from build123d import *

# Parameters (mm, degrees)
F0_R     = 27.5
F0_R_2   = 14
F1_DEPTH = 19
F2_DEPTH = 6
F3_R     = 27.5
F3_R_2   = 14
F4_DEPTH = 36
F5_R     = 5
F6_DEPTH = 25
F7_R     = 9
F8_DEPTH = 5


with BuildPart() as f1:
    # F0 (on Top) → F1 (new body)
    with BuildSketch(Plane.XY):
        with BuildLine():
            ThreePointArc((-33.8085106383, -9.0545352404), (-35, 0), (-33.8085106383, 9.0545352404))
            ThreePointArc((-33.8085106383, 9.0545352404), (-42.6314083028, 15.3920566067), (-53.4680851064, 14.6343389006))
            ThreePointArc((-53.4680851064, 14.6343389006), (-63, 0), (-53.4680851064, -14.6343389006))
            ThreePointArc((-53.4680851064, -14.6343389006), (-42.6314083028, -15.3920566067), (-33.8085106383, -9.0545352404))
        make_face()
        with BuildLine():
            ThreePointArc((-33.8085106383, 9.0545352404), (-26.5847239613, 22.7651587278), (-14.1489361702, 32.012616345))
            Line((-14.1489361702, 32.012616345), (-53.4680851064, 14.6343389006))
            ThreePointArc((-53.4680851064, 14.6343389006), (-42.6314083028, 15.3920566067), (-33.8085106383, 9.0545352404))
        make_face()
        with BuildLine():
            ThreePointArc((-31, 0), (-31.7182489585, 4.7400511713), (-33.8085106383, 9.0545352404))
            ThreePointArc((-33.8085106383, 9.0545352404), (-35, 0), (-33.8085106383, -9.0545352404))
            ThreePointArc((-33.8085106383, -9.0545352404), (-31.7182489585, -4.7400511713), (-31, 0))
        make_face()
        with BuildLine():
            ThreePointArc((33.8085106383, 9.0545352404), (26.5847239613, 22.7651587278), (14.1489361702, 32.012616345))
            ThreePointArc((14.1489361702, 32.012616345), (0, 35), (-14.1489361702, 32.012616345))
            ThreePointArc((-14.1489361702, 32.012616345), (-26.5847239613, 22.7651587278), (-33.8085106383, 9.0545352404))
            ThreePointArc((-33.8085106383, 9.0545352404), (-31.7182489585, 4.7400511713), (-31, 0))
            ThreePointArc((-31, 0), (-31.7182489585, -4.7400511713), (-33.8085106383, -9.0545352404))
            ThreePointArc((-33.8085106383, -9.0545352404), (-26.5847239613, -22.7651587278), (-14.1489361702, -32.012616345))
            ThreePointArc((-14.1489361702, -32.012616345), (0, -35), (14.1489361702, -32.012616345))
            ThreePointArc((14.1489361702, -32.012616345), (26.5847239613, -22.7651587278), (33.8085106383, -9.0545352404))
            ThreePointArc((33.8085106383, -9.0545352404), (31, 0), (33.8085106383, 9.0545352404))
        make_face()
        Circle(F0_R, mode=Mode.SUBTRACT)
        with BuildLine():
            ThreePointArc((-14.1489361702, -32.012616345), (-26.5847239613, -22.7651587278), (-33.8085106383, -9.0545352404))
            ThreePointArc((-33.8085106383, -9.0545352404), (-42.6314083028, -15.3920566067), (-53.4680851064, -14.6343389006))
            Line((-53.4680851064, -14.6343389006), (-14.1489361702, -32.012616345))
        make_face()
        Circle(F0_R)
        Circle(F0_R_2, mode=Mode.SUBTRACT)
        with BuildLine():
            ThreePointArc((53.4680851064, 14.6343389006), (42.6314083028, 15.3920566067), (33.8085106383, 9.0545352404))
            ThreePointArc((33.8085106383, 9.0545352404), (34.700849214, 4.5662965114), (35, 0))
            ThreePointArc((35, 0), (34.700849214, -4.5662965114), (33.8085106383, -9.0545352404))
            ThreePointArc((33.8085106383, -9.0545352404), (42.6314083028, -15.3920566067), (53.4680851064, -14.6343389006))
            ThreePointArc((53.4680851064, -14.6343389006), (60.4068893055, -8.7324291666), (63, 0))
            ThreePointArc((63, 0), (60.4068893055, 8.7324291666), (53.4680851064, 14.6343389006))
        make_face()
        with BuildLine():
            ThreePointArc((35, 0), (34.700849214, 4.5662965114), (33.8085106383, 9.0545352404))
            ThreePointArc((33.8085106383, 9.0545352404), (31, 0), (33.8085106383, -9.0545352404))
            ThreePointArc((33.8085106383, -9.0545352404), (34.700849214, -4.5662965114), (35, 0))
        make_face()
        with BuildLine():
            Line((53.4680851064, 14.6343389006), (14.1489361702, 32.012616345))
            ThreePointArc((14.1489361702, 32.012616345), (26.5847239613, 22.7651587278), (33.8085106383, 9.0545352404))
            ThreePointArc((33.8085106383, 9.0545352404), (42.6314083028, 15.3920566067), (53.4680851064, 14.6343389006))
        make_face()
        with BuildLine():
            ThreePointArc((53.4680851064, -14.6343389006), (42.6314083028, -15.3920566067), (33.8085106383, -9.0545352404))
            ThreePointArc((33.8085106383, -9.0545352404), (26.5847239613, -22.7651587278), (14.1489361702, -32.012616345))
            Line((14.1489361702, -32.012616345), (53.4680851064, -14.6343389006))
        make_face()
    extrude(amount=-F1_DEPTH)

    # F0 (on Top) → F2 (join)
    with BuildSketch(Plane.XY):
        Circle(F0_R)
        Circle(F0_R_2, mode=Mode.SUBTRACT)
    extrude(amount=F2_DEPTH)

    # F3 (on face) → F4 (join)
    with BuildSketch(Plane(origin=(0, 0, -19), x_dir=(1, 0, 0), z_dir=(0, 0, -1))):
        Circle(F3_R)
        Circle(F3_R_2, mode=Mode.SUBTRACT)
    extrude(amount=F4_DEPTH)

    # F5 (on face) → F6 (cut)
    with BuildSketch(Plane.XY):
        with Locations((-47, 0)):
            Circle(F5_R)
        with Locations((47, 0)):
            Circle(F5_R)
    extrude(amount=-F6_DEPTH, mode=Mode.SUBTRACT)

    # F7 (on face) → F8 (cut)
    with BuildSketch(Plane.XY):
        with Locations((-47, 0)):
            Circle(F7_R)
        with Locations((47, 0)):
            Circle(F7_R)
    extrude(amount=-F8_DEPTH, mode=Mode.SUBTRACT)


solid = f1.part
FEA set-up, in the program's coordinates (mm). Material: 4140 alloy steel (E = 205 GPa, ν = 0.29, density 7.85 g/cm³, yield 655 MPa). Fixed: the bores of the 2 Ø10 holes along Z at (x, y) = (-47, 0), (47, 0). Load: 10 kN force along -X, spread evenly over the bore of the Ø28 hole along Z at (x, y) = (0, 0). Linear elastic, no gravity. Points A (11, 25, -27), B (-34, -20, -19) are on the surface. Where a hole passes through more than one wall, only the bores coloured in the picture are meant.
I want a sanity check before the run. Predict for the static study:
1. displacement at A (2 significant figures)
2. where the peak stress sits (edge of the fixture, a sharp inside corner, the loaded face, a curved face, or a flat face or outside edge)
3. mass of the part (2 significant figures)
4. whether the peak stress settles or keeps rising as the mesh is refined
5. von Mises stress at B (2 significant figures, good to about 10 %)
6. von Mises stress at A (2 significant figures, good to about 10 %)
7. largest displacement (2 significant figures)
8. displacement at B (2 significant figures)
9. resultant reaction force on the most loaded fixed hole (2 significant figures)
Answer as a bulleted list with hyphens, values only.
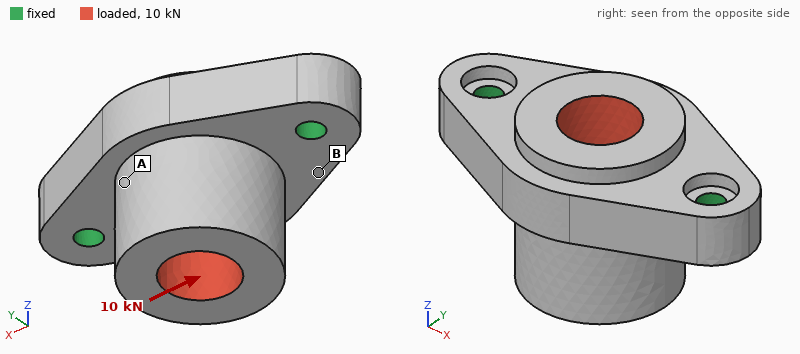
- 2.7 µm
- edge of the fixture
- 1.3 kg
- keeps rising
- 8.9 MPa
- 4.4 MPa
- 5.8 µm
- 1.4 µm
- 5.3 kN
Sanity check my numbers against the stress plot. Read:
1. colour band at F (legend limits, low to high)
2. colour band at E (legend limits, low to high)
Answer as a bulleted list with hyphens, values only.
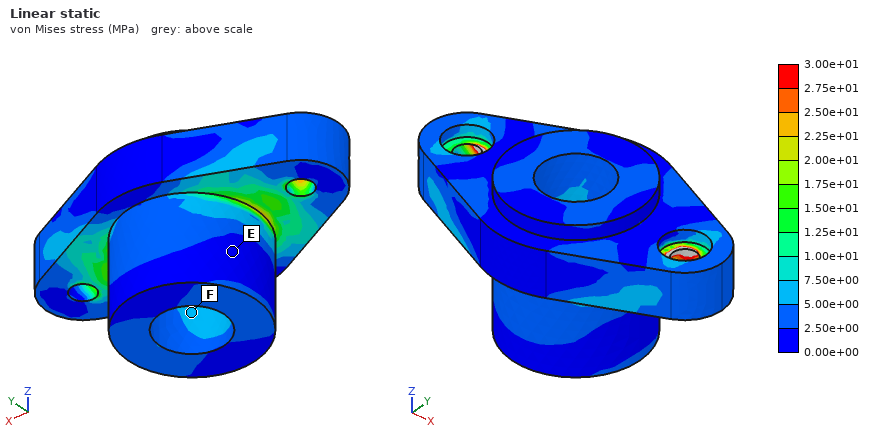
- 5.00e+00 to 7.50e+00 MPa
- 0.00e+00 to 2.50e+00 MPa
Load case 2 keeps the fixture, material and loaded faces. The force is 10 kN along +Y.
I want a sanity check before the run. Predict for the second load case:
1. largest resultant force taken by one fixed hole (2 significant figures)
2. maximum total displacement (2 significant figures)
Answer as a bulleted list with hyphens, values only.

- 5.0 kN
- 25 µm
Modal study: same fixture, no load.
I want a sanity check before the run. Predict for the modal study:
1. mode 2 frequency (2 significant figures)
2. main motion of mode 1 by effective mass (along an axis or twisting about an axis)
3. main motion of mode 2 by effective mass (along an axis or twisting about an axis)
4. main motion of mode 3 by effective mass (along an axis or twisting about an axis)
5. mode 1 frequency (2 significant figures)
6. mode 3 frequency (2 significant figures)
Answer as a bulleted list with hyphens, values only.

- 6000 Hz
- along Y
- along Z
- along X
- 3300 Hz
- 8100 Hz
